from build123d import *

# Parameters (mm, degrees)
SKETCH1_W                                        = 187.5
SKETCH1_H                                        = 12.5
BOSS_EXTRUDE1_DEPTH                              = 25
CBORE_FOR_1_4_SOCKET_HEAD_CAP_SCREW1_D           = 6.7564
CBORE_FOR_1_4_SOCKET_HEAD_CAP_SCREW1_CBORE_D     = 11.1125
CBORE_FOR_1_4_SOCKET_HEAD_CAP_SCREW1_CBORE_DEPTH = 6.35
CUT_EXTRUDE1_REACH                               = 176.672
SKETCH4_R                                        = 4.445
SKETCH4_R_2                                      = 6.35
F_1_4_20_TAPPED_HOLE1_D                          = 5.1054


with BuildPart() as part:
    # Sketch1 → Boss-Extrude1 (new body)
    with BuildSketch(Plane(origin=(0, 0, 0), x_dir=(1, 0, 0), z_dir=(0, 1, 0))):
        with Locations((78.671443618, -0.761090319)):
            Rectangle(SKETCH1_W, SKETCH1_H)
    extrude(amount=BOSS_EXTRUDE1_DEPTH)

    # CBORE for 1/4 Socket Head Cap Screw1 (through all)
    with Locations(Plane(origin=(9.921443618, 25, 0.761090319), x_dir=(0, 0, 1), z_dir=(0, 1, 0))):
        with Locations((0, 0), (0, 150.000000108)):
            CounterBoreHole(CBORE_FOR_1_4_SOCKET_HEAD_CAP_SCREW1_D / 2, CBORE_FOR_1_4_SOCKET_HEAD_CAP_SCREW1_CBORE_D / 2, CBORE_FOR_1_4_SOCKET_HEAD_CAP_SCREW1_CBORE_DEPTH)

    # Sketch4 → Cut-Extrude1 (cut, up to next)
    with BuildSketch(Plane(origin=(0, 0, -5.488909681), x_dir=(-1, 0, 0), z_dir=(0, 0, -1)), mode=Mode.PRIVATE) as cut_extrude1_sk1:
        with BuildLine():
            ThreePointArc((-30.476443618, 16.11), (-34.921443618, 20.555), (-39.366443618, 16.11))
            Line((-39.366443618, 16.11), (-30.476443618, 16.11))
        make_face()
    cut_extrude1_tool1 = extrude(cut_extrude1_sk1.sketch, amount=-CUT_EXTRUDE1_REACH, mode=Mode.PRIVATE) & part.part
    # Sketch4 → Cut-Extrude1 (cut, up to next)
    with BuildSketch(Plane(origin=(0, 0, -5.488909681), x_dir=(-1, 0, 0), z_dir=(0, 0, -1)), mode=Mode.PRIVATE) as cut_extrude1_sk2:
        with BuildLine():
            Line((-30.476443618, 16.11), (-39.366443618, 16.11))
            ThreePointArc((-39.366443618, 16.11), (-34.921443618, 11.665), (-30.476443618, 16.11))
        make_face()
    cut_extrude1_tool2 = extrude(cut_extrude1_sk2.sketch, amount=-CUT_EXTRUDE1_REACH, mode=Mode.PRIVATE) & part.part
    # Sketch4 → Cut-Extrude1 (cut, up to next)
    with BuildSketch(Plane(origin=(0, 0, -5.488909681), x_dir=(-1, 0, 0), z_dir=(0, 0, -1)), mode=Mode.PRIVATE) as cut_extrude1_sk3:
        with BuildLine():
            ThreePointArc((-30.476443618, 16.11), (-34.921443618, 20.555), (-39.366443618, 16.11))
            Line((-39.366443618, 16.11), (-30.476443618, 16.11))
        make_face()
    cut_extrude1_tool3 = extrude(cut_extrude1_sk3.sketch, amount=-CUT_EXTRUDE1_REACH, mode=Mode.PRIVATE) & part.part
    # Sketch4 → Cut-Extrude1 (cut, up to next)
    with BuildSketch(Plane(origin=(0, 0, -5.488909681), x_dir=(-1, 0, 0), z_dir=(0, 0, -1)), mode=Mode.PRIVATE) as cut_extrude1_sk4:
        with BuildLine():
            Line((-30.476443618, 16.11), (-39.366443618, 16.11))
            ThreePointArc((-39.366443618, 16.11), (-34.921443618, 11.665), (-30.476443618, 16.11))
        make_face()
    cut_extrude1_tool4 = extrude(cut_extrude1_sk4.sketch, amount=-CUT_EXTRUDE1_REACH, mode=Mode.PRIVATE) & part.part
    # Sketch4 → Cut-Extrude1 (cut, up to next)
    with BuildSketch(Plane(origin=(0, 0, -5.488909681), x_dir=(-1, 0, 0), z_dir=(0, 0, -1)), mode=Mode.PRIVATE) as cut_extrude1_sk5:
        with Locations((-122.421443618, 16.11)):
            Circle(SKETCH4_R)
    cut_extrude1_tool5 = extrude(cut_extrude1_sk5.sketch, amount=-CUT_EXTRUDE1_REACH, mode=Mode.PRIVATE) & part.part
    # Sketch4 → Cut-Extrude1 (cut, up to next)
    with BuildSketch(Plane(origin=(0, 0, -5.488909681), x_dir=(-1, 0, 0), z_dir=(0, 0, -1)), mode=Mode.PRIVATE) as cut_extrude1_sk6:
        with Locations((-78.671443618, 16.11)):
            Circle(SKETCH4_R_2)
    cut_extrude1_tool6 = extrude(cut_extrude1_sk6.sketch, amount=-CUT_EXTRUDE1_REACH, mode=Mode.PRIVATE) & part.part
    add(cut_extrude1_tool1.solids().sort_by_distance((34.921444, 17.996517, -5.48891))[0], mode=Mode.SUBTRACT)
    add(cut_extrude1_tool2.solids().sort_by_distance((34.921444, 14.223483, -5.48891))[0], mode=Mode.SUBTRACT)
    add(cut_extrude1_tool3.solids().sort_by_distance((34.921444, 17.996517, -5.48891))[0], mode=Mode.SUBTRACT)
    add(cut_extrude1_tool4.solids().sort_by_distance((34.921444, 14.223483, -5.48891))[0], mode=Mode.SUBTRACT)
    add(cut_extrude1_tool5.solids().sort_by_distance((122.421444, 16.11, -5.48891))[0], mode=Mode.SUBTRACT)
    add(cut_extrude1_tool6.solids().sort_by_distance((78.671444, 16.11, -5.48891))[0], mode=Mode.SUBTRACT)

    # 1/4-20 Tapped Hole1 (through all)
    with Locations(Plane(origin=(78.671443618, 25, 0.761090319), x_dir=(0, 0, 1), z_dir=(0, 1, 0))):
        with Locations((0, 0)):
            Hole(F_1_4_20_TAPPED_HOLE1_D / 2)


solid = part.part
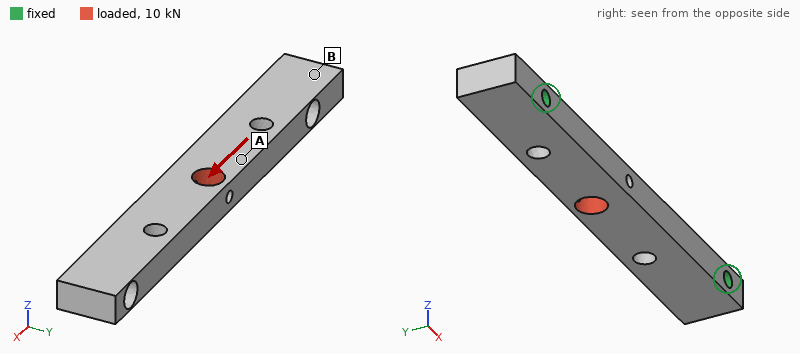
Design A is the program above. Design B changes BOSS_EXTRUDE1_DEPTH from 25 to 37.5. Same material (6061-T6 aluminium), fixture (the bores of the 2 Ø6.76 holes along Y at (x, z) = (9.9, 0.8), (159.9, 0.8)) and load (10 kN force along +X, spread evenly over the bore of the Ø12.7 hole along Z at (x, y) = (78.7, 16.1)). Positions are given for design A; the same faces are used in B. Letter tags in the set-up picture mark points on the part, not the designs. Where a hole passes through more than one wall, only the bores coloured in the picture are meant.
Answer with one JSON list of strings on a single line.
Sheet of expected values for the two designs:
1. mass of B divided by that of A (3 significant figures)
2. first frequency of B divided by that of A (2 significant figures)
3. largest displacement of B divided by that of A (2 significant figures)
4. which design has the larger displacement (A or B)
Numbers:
["1.51", "0.91", "0.74", "A"]
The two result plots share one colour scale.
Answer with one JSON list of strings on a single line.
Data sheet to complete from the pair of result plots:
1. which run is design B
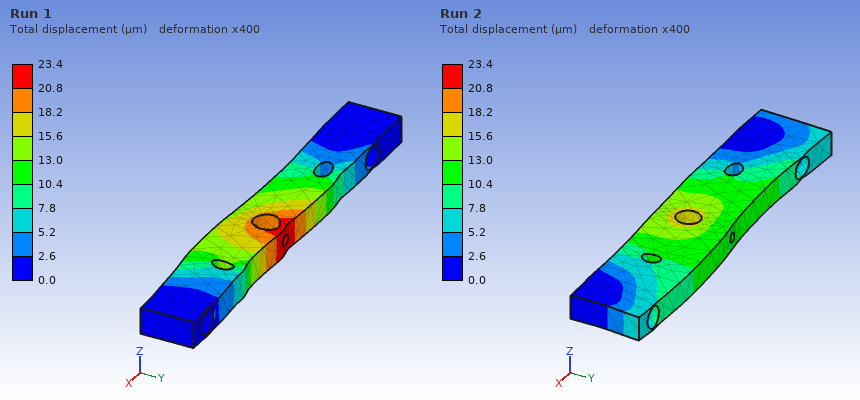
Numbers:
["Run 2"]
